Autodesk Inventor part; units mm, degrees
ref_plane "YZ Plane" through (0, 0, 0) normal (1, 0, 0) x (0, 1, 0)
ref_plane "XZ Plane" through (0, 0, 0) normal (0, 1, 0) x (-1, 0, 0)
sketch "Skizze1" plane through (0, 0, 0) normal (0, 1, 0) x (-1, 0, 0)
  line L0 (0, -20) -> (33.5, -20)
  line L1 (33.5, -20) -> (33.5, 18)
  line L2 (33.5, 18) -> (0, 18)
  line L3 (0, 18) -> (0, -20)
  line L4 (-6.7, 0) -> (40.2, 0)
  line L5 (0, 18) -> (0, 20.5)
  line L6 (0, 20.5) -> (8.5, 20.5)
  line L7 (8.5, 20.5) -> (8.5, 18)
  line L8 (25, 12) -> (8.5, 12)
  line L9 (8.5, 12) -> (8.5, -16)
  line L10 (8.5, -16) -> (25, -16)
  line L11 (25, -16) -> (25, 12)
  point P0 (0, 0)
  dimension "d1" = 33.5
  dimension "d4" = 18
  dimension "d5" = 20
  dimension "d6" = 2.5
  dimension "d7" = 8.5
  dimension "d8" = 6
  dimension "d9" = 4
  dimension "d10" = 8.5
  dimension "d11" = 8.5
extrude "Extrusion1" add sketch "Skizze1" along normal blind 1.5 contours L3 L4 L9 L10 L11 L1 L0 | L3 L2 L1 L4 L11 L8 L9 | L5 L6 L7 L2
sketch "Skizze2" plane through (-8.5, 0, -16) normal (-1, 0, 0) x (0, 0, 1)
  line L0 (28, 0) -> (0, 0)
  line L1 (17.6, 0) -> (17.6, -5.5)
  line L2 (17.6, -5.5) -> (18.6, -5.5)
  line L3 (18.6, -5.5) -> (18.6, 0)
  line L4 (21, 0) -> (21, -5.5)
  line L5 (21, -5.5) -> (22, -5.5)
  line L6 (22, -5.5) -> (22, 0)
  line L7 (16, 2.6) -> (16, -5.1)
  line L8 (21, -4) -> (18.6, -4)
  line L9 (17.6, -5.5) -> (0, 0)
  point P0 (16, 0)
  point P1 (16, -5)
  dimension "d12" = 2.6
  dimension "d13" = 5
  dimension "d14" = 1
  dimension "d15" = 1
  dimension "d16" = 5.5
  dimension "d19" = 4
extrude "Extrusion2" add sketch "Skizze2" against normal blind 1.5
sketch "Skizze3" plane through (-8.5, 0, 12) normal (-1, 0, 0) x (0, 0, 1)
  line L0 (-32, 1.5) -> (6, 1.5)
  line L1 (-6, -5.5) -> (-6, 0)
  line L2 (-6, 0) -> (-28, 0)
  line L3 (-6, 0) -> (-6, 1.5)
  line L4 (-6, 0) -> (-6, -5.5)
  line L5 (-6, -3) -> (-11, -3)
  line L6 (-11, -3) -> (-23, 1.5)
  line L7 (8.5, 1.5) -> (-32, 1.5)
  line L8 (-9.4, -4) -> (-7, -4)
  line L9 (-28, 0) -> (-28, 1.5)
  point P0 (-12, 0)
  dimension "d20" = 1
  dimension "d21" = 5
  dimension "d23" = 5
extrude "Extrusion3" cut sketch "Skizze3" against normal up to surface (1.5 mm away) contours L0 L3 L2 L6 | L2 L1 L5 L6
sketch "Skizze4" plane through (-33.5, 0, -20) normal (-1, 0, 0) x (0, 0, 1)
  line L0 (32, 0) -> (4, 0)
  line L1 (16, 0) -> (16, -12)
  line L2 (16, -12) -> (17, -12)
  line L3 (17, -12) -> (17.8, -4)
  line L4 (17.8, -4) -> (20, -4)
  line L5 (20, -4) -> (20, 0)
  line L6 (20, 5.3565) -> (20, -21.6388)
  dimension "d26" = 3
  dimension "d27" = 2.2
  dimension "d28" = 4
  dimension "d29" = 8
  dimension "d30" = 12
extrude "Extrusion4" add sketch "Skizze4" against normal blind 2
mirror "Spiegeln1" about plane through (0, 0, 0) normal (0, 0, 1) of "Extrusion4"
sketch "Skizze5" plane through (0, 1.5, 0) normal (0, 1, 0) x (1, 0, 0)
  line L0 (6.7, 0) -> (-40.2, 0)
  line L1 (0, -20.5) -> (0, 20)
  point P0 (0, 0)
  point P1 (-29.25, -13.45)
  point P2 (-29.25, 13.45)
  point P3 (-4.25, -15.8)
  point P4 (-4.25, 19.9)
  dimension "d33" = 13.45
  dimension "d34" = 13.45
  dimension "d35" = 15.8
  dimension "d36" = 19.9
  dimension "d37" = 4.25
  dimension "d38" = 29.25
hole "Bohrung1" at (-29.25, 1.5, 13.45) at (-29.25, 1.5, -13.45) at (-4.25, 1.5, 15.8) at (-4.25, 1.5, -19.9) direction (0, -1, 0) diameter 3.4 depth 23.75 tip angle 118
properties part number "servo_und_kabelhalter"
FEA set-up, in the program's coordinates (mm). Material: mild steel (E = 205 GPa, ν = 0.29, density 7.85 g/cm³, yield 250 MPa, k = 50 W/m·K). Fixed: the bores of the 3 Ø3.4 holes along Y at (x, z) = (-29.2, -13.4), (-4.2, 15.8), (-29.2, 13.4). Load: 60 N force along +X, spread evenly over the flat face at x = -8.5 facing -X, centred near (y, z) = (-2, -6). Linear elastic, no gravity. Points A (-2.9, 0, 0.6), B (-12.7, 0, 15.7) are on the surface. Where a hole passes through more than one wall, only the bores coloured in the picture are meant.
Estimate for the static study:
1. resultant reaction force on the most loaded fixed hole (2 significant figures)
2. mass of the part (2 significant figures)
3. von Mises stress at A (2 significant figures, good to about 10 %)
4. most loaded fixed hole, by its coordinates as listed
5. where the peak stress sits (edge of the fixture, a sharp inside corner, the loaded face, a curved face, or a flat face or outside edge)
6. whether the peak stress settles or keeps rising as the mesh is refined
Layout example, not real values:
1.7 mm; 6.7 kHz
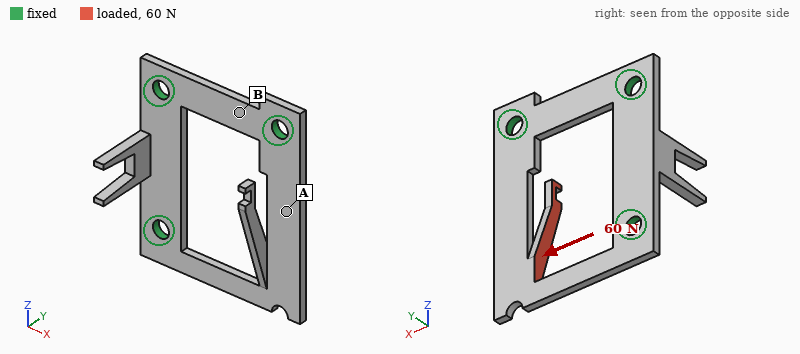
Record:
32 N; 11 g; 42 MPa; (-29.2, -13.4); a sharp inside corner; keeps rising
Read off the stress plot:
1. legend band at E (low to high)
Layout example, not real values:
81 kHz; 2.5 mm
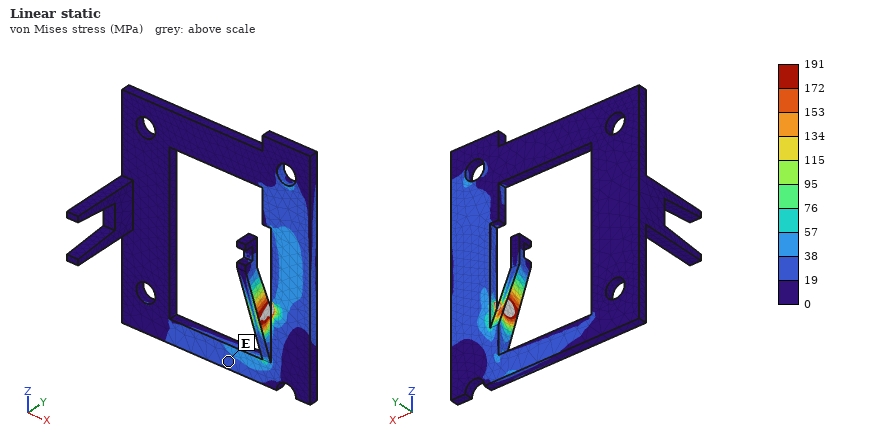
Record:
19 to 38 MPa
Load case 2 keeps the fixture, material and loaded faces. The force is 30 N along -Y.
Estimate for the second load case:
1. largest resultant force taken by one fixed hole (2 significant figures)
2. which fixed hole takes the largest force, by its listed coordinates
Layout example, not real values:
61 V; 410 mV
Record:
20 N; (-4.2, 15.8)
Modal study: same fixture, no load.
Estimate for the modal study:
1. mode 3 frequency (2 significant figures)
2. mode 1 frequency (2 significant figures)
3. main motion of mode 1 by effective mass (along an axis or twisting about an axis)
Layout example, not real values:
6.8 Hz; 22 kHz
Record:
5400 Hz; 1800 Hz; along Y
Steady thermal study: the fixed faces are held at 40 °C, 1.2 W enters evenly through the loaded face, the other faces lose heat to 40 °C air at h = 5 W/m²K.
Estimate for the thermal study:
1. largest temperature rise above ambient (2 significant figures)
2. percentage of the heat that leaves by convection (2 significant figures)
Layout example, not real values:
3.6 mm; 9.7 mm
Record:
68 K; 8.7 %
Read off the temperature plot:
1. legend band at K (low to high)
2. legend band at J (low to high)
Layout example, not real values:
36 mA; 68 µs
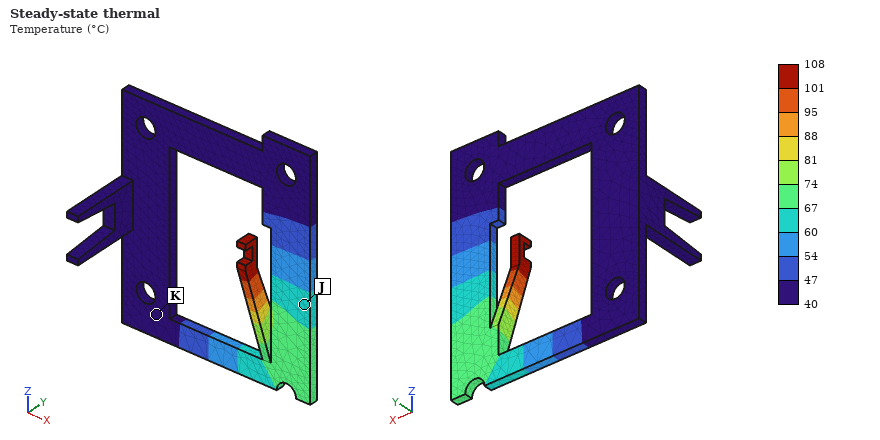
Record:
40 to 47 °C; 60 to 67 °C
